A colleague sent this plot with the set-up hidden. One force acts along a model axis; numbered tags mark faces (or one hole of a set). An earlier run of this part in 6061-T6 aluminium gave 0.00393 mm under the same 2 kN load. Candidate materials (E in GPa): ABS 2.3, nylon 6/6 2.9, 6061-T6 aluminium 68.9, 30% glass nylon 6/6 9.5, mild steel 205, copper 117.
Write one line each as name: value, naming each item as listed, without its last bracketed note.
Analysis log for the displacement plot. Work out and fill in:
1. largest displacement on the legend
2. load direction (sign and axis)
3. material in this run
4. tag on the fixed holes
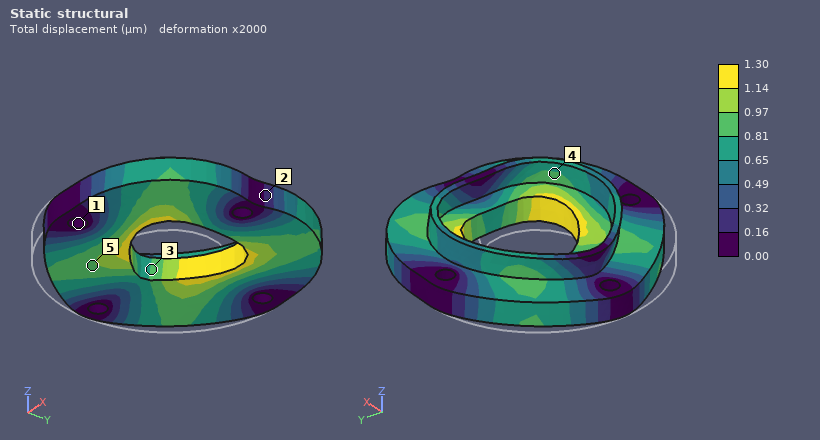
largest displacement on the legend: 1.30 µm
load direction: +X
material in this run: mild steel
tag on the fixed holes: 1
